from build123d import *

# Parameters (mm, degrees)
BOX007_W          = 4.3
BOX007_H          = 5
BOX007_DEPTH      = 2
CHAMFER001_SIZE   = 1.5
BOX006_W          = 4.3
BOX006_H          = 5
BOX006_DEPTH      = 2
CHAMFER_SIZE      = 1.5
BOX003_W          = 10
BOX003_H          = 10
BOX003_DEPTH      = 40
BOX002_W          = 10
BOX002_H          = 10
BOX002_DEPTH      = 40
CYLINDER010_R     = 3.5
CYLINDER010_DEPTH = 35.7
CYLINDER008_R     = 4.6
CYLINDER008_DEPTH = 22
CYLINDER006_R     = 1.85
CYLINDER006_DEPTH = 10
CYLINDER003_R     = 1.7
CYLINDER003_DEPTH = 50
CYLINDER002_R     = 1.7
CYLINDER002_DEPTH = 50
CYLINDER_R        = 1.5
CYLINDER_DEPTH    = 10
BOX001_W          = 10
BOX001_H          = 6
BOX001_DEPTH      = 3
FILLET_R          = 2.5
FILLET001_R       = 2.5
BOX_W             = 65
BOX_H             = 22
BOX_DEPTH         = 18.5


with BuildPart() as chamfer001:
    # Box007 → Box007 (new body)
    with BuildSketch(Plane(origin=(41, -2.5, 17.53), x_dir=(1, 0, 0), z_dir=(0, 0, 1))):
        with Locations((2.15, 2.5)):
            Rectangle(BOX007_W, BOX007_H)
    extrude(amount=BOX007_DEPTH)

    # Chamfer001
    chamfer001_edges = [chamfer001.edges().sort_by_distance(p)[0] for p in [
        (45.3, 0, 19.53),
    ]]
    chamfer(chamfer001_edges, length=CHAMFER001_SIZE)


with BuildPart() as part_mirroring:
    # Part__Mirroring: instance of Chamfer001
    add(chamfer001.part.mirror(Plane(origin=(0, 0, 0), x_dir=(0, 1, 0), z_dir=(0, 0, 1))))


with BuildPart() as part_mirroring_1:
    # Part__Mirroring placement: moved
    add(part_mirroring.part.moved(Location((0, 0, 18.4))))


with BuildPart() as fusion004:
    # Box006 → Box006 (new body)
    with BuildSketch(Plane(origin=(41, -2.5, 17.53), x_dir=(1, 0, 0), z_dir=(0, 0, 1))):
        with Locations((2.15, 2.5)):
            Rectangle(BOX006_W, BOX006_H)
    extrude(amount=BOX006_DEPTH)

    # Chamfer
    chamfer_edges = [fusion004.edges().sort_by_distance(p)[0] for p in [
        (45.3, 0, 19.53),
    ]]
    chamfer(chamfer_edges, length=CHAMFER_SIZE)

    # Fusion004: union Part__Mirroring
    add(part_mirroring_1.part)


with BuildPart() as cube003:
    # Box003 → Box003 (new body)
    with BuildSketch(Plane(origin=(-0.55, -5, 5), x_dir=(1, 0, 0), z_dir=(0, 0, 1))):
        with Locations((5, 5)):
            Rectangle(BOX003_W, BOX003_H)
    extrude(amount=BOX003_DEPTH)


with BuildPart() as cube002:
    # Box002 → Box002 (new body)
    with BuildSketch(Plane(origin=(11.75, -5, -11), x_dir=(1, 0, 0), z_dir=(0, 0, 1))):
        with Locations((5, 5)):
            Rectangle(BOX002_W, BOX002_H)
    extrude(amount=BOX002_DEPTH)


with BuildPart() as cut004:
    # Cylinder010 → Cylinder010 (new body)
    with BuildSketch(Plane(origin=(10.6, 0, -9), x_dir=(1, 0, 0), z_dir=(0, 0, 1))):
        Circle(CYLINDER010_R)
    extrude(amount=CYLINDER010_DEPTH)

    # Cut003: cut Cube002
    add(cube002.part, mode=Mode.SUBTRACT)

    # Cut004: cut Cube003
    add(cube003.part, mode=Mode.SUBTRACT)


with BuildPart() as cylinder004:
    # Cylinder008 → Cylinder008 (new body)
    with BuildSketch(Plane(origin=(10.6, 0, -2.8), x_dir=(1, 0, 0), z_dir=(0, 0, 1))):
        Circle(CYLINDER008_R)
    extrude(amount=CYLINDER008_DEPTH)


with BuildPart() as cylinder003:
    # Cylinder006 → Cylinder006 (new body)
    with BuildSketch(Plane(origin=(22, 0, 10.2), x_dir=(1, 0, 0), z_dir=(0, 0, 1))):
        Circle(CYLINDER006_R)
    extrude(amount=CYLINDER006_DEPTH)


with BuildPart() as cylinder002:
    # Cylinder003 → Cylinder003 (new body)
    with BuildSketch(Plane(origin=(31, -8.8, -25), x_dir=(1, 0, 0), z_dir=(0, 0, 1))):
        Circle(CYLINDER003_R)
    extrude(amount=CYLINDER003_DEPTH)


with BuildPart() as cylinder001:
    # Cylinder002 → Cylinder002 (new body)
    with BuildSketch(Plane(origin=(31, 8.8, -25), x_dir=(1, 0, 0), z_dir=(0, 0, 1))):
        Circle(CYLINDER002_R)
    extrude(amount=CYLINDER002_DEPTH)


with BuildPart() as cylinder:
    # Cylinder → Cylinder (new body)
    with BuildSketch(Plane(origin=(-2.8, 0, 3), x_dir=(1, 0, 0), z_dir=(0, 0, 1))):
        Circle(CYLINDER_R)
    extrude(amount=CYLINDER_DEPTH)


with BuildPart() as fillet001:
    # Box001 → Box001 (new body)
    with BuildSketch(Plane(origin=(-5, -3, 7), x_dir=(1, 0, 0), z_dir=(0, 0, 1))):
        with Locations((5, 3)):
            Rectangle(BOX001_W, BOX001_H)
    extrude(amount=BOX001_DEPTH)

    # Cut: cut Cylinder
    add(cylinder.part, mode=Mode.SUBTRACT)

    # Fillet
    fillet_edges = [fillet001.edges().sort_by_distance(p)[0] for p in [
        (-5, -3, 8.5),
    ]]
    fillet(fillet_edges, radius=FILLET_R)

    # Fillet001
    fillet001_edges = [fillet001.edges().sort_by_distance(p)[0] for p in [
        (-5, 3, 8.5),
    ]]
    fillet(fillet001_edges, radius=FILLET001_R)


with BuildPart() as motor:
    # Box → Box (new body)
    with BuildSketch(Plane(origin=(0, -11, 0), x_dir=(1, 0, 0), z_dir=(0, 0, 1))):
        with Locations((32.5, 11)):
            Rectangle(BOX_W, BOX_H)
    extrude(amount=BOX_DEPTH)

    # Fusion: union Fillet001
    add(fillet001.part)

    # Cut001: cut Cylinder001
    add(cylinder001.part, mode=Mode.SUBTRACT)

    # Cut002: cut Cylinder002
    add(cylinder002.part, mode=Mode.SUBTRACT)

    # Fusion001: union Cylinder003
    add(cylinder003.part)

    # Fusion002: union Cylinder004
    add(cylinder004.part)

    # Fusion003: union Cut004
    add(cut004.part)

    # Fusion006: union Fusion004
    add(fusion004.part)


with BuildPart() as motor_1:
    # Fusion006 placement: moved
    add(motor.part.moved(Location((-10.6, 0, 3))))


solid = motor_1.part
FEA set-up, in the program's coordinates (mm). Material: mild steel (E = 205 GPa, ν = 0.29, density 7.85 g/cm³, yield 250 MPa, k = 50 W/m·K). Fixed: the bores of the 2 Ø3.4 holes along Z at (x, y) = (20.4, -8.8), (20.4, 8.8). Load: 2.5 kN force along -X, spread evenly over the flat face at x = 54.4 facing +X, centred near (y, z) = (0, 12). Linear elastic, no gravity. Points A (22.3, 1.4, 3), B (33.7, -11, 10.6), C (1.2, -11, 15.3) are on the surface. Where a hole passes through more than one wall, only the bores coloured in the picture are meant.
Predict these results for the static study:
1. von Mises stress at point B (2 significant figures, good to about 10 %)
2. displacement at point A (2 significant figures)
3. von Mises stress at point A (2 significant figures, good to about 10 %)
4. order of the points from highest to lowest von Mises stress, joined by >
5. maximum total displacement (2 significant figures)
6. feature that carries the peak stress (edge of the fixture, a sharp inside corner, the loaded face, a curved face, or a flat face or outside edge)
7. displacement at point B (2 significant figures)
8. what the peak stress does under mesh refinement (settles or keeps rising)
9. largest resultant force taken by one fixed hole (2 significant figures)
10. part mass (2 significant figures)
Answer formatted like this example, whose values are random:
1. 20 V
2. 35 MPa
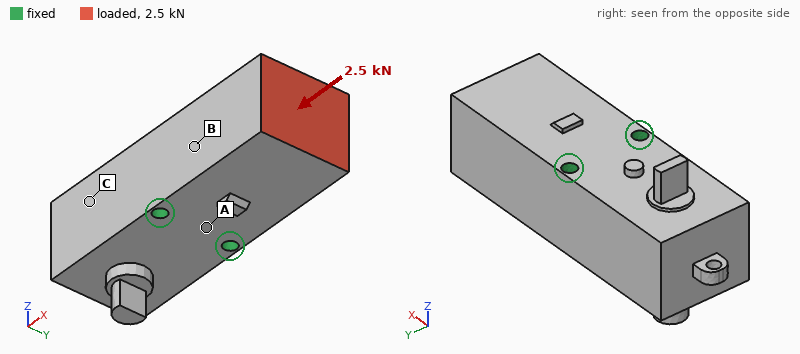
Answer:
1. 6.5 MPa
2. 0.21 µm
3. 2.7 MPa
4. B > A > C
5. 1.1 µm
6. edge of the fixture
7. 0.44 µm
8. keeps rising
9. 1.3 kN
10. 210 g
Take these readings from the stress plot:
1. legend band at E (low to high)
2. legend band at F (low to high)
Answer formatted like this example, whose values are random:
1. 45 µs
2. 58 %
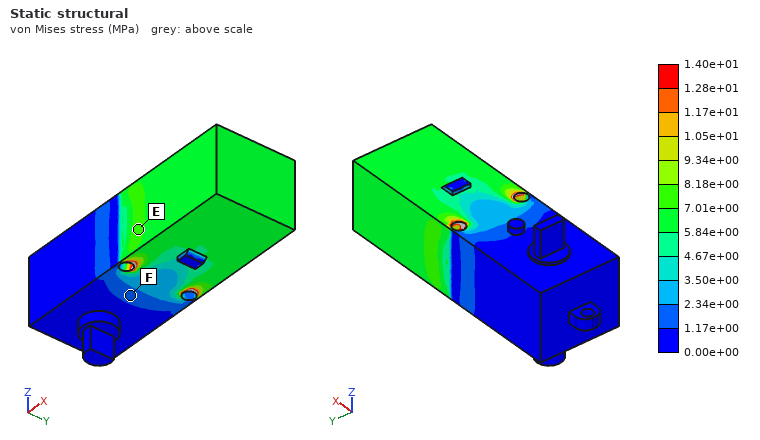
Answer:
1. 7.01e+00 to 8.18e+00 MPa
2. 1.17e+00 to 2.34e+00 MPa
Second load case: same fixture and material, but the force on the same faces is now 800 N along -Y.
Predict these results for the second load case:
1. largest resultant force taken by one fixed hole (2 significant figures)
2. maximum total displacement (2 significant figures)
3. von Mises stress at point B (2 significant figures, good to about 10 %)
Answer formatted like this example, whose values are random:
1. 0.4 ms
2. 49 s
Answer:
1. 1.5 kN
2. 4.1 µm
3. 11 MPa
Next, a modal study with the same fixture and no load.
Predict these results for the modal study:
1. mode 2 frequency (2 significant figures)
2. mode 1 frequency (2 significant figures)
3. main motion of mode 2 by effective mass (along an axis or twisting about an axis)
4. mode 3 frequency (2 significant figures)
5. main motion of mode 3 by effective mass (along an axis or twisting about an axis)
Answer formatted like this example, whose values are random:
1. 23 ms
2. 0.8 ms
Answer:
1. 12 kHz
2. 10 kHz
3. along Z
4. 13 kHz
5. along Y
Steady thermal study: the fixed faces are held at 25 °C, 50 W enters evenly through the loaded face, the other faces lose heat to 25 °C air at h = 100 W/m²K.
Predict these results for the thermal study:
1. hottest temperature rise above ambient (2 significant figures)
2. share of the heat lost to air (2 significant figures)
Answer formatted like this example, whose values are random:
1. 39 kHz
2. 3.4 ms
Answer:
1. 74 K
2. 21 %
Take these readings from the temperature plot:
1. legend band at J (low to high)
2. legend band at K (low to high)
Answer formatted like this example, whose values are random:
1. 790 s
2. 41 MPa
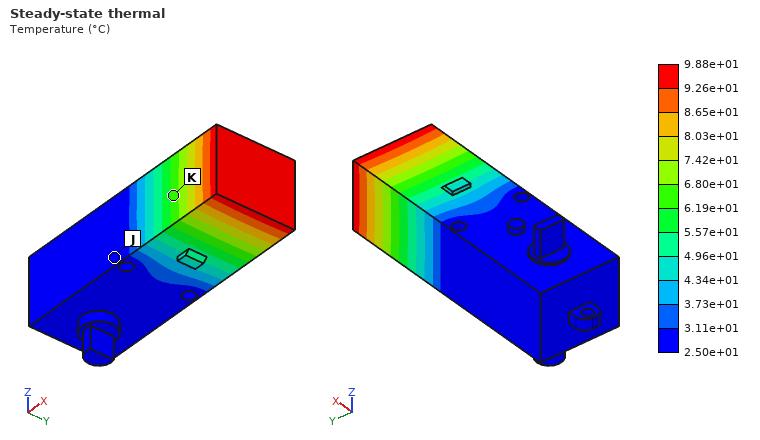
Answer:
1. 2.50e+01 to 3.11e+01 °C
2. 6.19e+01 to 6.80e+01 °C
